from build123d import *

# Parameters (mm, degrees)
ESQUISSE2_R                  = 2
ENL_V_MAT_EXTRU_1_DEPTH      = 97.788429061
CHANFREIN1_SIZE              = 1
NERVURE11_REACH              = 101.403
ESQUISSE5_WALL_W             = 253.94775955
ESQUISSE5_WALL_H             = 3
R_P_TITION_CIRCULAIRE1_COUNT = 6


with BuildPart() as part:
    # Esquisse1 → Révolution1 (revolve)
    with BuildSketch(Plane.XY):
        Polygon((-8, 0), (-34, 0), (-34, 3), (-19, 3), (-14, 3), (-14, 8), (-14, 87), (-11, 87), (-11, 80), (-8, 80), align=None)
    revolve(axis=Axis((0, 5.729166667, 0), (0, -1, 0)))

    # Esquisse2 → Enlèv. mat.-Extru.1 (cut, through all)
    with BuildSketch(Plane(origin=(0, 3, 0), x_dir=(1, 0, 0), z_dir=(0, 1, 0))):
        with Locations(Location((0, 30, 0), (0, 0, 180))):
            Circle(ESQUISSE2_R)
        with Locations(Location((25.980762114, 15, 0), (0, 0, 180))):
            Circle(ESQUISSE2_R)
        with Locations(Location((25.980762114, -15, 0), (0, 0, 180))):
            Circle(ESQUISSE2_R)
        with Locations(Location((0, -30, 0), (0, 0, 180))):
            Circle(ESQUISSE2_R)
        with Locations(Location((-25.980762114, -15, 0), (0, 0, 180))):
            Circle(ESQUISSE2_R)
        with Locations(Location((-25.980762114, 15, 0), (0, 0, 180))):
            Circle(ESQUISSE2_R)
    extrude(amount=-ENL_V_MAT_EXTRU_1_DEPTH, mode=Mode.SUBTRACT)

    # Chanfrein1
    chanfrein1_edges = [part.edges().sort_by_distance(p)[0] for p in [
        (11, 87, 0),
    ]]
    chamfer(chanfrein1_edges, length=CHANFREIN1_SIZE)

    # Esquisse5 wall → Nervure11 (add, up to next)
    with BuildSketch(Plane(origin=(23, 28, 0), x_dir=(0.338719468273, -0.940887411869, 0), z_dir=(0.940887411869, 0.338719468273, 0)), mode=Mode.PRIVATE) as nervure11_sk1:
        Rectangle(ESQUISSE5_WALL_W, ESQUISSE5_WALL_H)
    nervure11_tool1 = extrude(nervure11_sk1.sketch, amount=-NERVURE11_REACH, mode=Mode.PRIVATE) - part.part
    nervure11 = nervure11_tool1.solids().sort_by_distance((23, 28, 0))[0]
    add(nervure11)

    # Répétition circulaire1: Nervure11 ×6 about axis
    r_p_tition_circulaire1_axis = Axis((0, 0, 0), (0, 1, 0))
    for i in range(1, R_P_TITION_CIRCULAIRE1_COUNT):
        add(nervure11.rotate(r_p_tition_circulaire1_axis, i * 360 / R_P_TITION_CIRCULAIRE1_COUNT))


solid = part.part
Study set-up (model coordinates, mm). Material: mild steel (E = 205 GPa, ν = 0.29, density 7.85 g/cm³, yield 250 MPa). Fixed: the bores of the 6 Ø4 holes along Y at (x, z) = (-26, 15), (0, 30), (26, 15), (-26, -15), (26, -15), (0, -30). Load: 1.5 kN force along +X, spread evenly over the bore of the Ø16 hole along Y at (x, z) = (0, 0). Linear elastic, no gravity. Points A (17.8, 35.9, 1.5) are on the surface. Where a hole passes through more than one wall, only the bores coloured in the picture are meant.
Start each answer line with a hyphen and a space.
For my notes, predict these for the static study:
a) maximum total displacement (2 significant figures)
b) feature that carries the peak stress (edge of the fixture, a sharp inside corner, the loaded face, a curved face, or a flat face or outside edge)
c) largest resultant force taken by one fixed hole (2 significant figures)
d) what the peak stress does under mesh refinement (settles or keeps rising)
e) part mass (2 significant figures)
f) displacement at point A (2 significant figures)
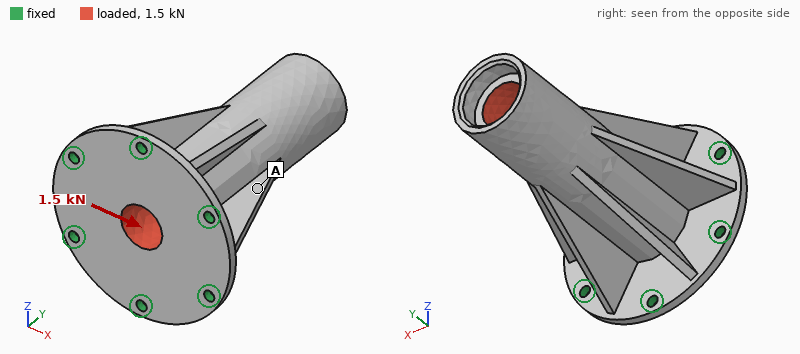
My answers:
- 47 µm
- edge of the fixture
- 660 N
- keeps rising
- 410 g
- 20 µm
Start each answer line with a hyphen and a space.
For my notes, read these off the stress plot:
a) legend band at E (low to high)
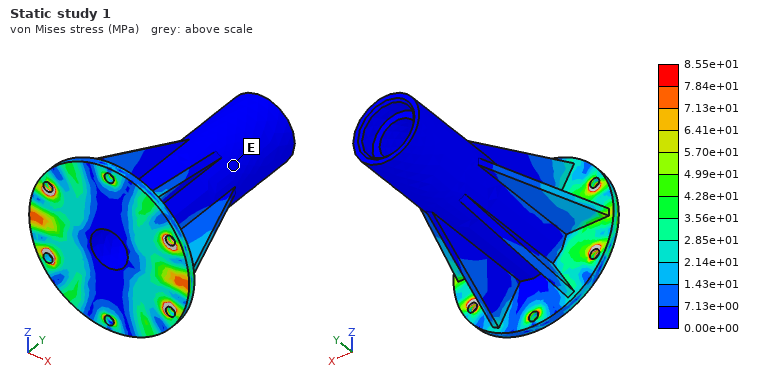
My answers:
- 0.00e+00 to 7.13e+00 MPa
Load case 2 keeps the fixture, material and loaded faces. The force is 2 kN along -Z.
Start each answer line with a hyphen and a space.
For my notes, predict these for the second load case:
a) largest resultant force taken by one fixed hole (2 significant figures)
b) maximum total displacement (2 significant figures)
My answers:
- 1.0 kN
- 63 µm
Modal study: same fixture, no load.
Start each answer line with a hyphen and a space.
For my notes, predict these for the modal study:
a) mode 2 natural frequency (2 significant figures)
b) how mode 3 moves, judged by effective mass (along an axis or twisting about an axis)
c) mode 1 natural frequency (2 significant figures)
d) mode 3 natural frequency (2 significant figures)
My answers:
- 2000 Hz
- along Y
- 2000 Hz
- 4800 Hz
